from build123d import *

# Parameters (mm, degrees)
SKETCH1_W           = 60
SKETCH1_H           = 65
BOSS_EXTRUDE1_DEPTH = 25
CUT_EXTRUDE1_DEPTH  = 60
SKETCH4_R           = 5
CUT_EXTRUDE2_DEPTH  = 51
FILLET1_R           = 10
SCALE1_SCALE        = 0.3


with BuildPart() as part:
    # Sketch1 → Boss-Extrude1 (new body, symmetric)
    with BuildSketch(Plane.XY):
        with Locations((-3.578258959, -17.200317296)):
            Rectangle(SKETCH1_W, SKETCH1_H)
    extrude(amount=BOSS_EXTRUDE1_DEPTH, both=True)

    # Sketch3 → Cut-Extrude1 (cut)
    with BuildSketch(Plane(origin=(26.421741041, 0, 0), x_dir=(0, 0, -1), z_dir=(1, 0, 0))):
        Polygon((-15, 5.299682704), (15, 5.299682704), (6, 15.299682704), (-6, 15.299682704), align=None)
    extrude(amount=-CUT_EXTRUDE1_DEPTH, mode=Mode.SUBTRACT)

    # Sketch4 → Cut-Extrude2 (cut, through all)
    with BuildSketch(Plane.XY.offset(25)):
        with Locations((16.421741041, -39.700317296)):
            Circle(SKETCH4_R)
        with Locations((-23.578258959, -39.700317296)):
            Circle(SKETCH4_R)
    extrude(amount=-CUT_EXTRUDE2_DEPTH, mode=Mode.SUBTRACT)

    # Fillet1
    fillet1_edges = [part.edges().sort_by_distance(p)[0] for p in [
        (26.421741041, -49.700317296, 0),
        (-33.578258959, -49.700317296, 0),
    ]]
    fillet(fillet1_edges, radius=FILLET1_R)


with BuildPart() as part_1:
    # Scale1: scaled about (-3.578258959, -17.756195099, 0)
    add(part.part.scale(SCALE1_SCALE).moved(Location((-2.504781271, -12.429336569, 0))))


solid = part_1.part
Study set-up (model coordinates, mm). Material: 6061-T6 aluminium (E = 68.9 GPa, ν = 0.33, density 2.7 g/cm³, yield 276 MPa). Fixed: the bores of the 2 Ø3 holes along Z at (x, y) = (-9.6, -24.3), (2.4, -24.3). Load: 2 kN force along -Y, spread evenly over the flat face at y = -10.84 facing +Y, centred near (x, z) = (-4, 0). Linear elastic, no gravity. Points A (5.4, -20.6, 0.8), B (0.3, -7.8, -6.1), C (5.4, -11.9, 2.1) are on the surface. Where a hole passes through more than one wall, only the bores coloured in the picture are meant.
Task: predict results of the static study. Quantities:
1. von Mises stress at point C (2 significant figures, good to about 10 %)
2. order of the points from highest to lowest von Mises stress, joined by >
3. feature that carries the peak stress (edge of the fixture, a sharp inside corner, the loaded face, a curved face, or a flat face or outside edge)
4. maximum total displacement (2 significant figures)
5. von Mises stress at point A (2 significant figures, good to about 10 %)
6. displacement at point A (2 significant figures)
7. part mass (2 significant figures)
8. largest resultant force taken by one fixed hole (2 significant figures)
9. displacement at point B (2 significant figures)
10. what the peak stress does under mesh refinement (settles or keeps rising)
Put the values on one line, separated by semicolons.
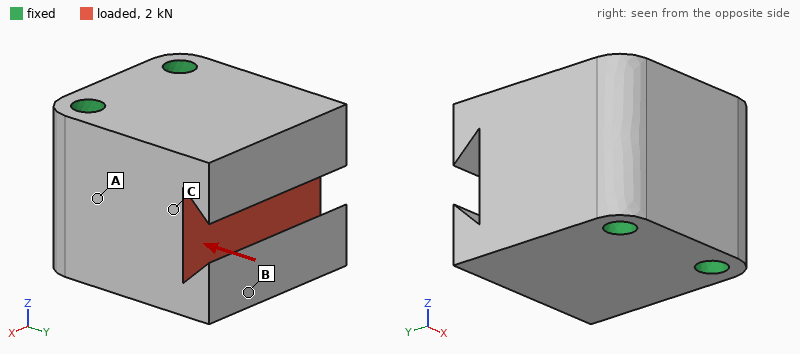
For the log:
12 MPa; C > A > B; edge of the fixture; 2.1 µm; 7.6 MPa; 0.53 µm; 13 g; 1.0 kN; 1.3 µm; keeps rising
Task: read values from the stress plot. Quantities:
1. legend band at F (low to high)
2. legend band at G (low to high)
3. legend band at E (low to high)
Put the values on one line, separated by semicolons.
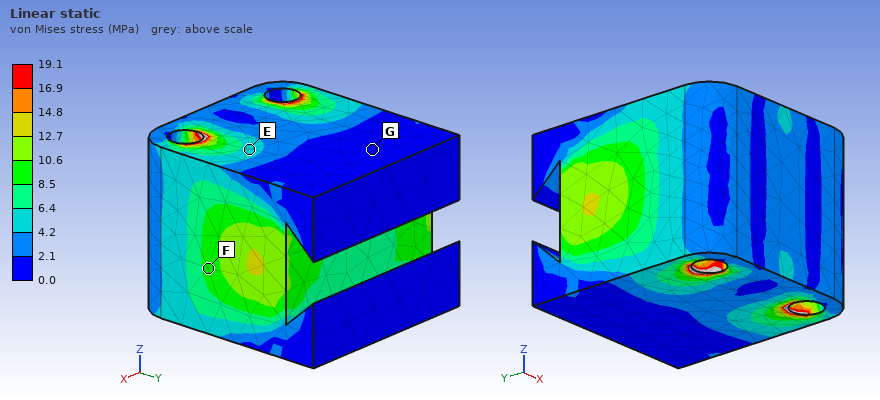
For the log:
8.5 to 10.6 MPa; 0.0 to 2.1 MPa; 4.2 to 6.4 MPa
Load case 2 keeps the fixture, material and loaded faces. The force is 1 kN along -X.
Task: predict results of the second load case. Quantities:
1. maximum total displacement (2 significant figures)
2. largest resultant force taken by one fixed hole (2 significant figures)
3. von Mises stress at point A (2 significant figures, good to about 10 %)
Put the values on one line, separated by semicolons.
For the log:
5.0 µm; 1.1 kN; 10 MPa
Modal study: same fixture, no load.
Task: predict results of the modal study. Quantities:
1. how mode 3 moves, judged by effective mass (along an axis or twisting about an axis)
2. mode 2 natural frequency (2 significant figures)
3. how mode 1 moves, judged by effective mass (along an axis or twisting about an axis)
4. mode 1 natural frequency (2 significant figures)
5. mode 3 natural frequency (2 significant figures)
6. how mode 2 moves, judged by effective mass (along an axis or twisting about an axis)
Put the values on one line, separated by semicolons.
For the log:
twisting about Y; 38 kHz; along Z; 32 kHz; 47 kHz; along X
